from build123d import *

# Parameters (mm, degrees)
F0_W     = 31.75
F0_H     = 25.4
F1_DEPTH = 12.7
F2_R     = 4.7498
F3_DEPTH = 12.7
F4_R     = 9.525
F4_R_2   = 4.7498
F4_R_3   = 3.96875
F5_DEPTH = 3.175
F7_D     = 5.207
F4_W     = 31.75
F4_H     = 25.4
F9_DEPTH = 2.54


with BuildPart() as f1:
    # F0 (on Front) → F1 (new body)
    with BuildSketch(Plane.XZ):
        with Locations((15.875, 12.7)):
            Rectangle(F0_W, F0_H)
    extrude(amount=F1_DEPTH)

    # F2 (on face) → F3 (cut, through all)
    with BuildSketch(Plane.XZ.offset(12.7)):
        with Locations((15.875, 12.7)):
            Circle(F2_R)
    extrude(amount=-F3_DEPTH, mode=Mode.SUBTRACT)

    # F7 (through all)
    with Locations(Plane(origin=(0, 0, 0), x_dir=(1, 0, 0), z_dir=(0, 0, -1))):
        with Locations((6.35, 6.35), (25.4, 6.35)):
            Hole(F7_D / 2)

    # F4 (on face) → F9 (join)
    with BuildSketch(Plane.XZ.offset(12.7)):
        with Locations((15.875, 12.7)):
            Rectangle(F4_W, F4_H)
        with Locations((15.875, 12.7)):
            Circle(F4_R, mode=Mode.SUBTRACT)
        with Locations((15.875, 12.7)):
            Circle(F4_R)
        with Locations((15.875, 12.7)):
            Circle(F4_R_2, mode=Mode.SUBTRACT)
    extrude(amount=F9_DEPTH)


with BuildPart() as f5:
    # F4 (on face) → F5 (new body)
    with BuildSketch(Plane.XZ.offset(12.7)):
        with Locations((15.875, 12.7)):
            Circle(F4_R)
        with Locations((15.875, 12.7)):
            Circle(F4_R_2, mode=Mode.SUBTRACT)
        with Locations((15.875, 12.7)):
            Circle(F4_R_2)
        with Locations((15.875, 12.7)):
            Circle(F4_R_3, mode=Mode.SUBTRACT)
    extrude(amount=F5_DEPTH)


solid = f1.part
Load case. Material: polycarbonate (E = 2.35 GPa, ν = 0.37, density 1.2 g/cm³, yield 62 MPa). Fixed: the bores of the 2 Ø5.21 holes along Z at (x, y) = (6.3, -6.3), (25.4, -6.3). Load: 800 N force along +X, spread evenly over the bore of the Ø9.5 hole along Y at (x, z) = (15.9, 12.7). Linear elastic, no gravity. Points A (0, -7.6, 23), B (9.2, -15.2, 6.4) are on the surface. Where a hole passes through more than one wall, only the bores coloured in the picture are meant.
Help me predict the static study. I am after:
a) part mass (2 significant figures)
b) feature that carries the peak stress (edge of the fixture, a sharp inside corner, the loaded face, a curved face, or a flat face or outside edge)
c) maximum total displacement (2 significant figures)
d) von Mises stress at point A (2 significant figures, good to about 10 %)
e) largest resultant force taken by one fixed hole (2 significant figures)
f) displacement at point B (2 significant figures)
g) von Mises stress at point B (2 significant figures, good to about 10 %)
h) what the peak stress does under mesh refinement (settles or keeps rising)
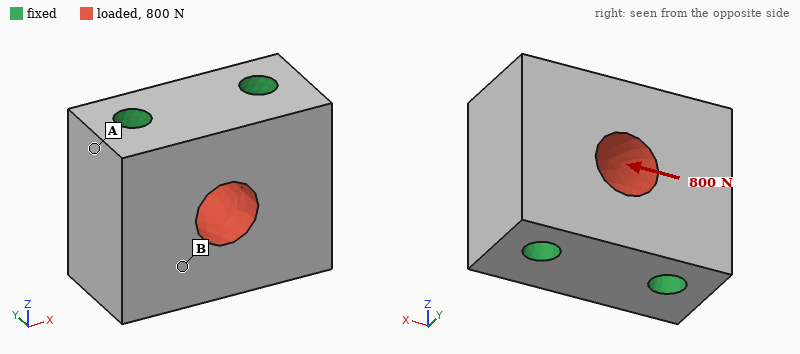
12 g
edge of the fixture
9.8 µm
0.54 MPa
400 N
4.8 µm
1.1 MPa
keeps rising
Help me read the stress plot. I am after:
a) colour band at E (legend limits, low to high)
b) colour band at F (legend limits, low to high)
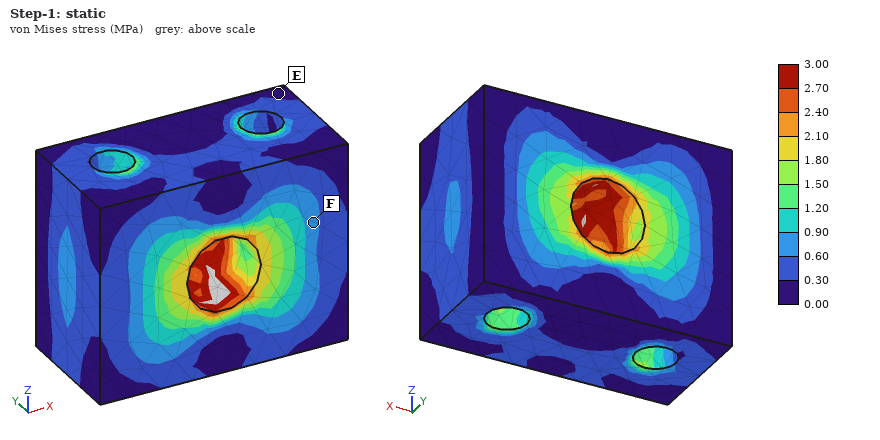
0.00 to 0.30 MPa
0.60 to 0.90 MPa
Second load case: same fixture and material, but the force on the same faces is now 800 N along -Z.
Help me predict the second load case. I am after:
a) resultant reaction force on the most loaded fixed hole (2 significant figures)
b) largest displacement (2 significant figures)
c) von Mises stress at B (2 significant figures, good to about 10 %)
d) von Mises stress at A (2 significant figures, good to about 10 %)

400 N
13 µm
1.3 MPa
0.41 MPa
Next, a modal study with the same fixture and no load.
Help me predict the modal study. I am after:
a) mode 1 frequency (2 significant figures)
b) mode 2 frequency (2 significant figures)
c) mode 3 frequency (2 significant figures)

20 kHz
21 kHz
21 kHz
